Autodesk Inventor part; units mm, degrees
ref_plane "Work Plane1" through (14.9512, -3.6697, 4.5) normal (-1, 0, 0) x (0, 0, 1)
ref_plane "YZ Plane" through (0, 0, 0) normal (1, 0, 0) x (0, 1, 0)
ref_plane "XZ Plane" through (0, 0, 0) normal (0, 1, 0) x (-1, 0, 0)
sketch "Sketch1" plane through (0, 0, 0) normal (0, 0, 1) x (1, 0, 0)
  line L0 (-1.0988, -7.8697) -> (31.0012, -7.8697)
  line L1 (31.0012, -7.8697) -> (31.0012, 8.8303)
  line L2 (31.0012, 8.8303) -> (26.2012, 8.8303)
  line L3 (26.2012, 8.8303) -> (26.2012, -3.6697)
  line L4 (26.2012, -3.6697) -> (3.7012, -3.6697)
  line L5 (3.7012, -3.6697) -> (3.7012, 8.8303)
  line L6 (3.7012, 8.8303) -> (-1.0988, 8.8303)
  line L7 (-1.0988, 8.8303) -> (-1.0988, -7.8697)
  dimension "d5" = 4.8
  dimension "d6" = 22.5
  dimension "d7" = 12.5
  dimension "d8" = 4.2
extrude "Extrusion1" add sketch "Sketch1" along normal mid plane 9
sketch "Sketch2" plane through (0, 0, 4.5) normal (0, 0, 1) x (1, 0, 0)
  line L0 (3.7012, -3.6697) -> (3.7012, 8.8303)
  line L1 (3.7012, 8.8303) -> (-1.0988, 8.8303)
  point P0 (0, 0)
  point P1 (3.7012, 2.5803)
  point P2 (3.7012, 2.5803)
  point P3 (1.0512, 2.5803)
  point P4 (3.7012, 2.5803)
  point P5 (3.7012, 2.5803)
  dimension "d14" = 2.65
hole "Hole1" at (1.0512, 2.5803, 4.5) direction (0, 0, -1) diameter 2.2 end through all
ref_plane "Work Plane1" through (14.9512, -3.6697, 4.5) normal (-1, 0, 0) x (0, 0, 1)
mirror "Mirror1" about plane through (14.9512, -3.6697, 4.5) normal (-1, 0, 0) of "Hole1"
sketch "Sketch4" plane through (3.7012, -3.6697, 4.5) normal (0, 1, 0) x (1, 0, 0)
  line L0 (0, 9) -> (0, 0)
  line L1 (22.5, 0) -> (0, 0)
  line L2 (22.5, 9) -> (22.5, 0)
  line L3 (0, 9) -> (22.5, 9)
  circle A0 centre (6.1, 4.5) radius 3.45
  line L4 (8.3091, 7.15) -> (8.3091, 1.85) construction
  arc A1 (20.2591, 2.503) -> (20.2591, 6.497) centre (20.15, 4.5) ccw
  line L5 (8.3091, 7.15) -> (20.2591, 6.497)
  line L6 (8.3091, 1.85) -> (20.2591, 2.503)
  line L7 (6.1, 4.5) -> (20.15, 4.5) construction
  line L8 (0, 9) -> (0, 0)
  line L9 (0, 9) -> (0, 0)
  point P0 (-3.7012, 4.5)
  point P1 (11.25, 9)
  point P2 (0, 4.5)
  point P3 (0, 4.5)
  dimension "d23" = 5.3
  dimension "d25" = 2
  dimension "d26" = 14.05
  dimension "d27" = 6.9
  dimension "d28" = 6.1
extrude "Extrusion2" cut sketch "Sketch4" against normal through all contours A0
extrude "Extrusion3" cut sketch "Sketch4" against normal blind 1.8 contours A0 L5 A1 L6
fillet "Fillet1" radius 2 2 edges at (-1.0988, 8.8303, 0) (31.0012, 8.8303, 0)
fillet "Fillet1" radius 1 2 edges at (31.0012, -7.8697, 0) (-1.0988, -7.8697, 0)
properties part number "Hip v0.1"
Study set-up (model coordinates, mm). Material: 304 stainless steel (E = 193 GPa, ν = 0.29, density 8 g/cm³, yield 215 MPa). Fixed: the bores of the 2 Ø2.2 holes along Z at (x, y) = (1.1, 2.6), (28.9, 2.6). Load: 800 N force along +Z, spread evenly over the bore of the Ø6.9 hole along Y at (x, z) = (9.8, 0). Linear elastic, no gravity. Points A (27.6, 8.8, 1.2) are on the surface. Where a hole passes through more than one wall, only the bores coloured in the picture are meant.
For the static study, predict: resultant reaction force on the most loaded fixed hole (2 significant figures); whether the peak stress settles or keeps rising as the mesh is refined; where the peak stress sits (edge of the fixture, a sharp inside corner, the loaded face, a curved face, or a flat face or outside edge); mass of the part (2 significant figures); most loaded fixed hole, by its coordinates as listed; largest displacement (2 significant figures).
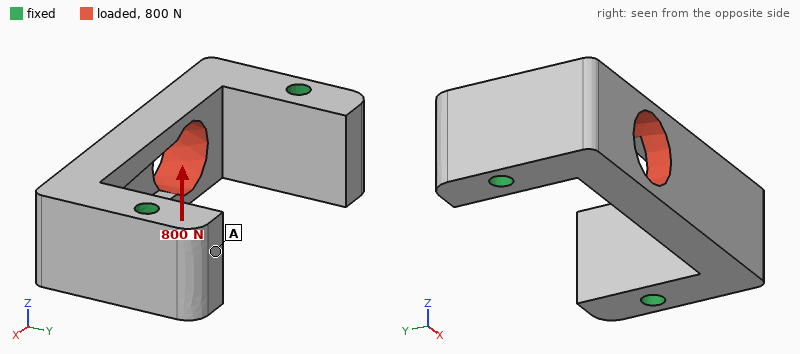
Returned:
550 N
keeps rising
edge of the fixture
16 g
(1.1, 2.6)
11 µm
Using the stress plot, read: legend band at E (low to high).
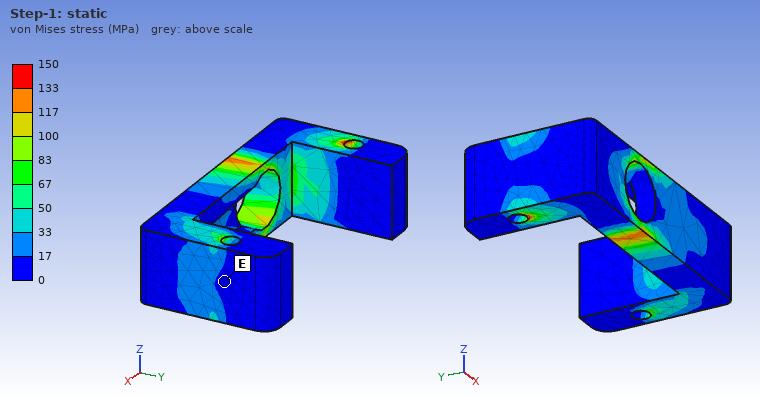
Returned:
0 to 17 MPa
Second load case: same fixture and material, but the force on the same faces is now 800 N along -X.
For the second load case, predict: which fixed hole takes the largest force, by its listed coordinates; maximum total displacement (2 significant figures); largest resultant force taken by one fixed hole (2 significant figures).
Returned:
(1.1, 2.6)
6.6 µm
430 N
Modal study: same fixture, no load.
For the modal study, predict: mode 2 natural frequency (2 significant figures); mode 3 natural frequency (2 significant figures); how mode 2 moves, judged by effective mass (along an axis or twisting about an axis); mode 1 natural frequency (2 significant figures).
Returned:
22 kHz
24 kHz
along X
21 kHz
